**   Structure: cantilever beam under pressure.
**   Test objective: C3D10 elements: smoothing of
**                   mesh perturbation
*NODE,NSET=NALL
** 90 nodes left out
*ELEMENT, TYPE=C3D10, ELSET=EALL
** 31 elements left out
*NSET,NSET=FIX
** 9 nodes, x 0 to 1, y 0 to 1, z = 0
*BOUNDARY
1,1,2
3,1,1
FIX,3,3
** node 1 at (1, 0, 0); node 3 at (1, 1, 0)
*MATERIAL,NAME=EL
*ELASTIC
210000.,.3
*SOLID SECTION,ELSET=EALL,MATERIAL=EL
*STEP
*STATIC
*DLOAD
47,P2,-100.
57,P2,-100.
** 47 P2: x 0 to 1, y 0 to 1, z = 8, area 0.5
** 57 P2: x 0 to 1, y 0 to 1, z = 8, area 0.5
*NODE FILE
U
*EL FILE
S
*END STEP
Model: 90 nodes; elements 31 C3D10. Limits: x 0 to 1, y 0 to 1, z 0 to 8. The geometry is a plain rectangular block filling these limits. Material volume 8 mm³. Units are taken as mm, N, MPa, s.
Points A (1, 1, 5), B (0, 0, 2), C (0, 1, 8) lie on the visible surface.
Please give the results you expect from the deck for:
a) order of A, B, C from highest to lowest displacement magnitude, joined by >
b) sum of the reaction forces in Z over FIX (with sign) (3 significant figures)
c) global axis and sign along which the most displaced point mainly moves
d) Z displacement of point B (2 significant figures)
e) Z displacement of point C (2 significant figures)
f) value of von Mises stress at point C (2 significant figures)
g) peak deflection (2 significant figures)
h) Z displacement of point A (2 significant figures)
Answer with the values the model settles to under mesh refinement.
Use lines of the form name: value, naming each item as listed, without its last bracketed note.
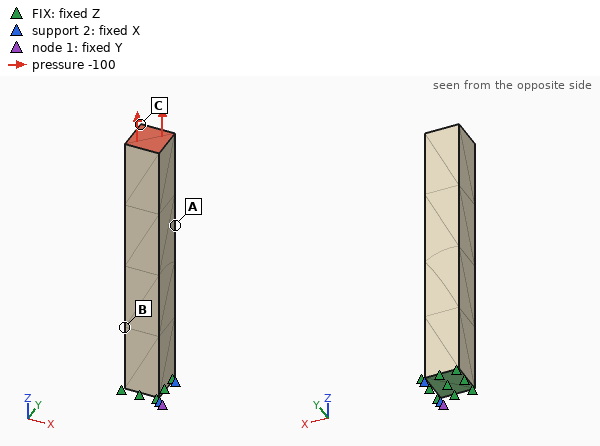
order of A, B, C from highest to lowest displacement magnitude, joined by >: C > A > B
sum of the reaction forces in Z over FIX (with sign): -100 N
global axis and sign along which the most displaced point mainly moves: +Z
Z displacement of point B: 9.5e-04 mm
Z displacement of point C: 0.0038 mm
value of von Mises stress at point C: 100 MPa
peak deflection: 0.0038 mm
Z displacement of point A: 0.0024 mm
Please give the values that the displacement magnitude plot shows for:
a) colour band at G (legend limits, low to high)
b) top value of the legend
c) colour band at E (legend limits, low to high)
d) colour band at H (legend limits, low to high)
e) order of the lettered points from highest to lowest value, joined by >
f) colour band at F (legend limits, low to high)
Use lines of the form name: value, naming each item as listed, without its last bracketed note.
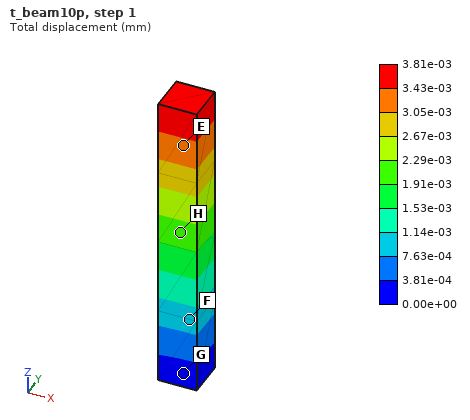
colour band at G: 0.00e+00 to 3.81e-04 mm
top value of the legend: 3.81e-03 mm
colour band at E: 3.05e-03 to 3.43e-03 mm
colour band at H: 1.91e-03 to 2.29e-03 mm
order of the lettered points from highest to lowest value, joined by >: E > H > F > G
colour band at F: 7.63e-04 to 1.14e-03 mm
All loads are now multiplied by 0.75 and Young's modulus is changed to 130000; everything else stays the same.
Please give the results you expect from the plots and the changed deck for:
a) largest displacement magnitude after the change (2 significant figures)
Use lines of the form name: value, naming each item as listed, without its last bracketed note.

largest displacement magnitude after the change: 0.0046 mm
